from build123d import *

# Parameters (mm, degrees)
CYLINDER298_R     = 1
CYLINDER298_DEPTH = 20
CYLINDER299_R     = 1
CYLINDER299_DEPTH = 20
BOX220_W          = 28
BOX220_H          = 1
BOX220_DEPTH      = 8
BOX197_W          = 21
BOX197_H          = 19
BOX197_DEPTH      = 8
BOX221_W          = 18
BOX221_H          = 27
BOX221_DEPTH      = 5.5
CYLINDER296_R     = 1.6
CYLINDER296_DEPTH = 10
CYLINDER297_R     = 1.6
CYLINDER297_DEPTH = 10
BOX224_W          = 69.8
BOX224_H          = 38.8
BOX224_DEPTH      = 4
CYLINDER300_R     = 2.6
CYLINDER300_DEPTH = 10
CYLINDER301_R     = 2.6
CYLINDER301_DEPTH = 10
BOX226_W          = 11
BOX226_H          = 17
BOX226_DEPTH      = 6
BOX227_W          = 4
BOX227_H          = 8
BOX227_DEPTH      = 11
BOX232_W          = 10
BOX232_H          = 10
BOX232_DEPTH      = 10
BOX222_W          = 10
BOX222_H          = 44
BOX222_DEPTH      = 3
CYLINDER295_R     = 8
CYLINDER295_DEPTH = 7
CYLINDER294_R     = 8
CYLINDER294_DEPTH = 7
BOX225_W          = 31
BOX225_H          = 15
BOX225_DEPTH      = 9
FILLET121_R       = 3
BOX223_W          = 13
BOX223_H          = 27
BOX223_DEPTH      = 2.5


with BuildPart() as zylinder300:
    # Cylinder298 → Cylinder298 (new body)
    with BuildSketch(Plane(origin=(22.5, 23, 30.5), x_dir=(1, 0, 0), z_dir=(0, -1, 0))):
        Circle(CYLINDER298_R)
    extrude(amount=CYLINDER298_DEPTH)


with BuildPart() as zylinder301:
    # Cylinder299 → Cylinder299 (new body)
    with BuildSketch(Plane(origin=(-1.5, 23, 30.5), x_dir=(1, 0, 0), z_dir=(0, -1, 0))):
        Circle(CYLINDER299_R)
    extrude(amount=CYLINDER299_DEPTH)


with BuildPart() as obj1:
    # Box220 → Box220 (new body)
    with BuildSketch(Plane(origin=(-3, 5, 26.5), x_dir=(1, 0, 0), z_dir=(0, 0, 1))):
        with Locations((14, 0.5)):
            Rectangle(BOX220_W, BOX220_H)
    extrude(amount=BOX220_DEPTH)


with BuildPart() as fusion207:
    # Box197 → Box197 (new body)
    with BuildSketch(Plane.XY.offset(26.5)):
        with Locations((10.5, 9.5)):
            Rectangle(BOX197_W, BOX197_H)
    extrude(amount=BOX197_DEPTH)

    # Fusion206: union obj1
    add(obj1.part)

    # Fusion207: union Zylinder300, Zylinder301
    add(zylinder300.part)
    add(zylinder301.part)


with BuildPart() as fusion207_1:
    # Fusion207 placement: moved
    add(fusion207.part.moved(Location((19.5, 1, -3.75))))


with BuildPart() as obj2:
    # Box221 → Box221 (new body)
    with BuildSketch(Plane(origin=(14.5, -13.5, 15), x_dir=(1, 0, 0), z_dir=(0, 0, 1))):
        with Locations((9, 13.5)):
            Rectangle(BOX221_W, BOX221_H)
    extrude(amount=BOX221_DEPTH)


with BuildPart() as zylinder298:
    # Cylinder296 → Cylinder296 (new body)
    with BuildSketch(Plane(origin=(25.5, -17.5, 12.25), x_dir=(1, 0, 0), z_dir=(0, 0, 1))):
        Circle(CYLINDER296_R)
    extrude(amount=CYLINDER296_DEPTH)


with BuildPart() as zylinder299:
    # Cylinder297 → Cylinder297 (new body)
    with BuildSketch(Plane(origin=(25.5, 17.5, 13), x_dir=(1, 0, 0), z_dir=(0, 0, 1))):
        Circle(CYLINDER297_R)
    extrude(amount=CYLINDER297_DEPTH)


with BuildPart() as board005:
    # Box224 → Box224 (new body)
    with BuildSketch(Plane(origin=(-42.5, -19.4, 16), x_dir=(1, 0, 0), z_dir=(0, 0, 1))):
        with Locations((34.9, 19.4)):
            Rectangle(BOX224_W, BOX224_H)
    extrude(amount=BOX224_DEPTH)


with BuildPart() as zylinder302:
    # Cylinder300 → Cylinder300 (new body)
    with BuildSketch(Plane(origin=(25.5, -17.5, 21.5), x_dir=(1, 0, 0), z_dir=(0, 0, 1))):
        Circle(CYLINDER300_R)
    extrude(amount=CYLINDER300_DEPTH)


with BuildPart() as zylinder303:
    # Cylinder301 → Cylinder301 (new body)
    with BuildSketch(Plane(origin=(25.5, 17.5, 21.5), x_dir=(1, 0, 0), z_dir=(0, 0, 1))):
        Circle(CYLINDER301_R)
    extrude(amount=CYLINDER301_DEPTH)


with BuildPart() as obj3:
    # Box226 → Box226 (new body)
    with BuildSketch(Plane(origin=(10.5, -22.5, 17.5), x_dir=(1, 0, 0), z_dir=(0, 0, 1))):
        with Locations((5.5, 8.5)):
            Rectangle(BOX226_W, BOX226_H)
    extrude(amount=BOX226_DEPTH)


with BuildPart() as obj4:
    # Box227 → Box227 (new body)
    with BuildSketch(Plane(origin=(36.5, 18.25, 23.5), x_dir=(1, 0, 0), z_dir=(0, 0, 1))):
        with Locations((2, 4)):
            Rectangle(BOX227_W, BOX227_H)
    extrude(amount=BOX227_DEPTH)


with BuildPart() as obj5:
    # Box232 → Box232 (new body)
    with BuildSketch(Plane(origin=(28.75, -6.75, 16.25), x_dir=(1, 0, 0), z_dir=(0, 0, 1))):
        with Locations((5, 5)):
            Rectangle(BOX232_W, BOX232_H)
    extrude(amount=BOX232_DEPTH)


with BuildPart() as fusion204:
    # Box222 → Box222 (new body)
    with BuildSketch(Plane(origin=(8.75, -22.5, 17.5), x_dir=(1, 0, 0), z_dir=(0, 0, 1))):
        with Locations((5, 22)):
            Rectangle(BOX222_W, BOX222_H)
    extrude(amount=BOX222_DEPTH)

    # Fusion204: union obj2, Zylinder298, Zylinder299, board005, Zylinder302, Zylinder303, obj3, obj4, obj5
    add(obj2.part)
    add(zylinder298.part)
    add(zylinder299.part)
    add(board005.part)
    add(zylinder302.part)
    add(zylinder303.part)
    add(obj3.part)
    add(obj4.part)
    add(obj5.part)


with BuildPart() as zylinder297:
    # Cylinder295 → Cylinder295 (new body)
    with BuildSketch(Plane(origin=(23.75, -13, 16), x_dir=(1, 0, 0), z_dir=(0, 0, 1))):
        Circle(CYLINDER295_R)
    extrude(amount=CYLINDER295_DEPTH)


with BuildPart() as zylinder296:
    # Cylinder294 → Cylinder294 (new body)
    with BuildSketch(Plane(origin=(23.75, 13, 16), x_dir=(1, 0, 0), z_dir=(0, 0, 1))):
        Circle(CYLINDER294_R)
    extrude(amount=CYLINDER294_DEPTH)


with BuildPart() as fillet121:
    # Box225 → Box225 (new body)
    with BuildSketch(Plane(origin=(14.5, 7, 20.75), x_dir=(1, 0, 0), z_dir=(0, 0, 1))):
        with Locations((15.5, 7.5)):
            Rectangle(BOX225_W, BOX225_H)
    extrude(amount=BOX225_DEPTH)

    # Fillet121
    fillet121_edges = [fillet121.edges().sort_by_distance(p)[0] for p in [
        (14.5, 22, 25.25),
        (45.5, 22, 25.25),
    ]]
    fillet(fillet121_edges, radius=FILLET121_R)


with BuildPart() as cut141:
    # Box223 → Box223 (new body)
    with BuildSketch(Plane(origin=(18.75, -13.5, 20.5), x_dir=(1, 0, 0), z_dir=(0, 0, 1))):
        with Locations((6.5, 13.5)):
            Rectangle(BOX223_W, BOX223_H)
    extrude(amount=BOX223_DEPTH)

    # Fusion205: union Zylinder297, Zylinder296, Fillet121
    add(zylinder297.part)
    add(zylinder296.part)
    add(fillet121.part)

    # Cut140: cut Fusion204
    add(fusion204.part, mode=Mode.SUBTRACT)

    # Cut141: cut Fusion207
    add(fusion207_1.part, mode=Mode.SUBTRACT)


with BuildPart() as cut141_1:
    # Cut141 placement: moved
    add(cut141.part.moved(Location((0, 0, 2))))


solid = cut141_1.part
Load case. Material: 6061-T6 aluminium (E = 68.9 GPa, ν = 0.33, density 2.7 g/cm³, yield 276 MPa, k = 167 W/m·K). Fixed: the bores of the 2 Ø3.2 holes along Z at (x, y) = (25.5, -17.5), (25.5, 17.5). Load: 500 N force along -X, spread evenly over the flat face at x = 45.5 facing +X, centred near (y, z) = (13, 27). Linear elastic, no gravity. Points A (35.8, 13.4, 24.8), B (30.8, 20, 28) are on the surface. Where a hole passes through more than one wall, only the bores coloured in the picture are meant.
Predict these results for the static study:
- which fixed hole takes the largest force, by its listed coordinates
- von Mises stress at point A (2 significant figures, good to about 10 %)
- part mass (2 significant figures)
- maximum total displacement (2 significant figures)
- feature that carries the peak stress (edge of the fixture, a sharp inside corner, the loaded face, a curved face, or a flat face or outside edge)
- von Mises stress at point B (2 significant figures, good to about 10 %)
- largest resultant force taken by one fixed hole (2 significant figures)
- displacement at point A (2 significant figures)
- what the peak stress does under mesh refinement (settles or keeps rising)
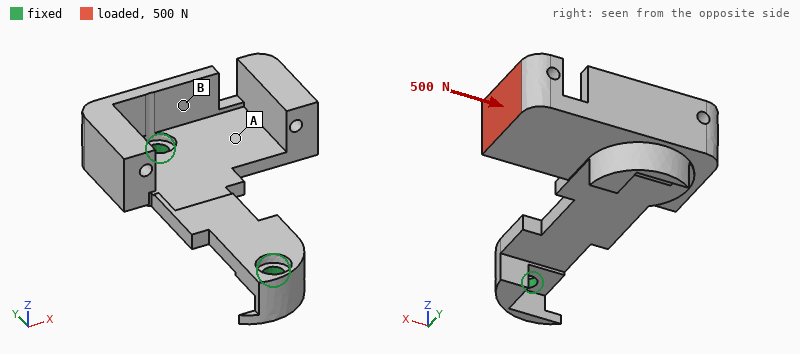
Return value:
(25.5, 17.5)
110 MPa
8.2 g
0.31 mm
edge of the fixture
23 MPa
430 N
0.060 mm
keeps rising
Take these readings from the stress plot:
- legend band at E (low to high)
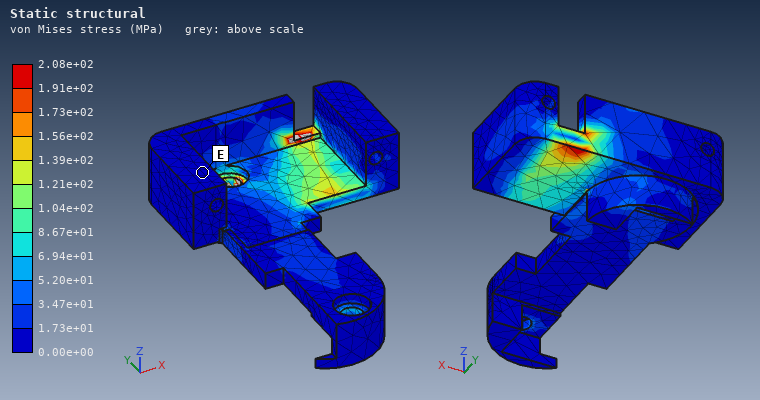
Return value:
0.00e+00 to 1.73e+01 MPa
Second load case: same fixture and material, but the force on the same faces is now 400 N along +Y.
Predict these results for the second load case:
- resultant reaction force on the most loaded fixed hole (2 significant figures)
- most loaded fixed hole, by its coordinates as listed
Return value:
380 N
(25.5, 17.5)
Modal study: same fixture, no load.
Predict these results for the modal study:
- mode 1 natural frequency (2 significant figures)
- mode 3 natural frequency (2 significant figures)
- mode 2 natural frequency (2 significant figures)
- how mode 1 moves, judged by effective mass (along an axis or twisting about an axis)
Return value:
3200 Hz
8800 Hz
6000 Hz
along Z
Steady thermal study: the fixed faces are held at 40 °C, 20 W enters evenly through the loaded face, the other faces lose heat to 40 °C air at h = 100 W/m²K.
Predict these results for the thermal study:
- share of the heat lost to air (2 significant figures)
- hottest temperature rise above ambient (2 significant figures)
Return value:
23 %
58 K
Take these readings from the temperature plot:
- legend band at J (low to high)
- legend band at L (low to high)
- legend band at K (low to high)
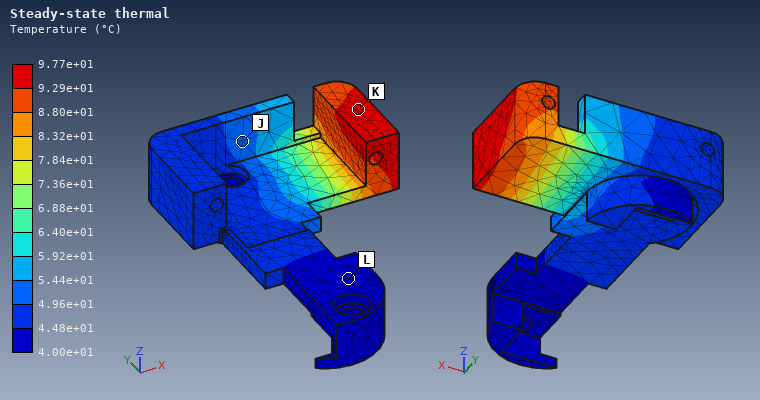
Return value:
4.96e+01 to 5.44e+01 °C
4.00e+01 to 4.48e+01 °C
9.29e+01 to 9.77e+01 °C
